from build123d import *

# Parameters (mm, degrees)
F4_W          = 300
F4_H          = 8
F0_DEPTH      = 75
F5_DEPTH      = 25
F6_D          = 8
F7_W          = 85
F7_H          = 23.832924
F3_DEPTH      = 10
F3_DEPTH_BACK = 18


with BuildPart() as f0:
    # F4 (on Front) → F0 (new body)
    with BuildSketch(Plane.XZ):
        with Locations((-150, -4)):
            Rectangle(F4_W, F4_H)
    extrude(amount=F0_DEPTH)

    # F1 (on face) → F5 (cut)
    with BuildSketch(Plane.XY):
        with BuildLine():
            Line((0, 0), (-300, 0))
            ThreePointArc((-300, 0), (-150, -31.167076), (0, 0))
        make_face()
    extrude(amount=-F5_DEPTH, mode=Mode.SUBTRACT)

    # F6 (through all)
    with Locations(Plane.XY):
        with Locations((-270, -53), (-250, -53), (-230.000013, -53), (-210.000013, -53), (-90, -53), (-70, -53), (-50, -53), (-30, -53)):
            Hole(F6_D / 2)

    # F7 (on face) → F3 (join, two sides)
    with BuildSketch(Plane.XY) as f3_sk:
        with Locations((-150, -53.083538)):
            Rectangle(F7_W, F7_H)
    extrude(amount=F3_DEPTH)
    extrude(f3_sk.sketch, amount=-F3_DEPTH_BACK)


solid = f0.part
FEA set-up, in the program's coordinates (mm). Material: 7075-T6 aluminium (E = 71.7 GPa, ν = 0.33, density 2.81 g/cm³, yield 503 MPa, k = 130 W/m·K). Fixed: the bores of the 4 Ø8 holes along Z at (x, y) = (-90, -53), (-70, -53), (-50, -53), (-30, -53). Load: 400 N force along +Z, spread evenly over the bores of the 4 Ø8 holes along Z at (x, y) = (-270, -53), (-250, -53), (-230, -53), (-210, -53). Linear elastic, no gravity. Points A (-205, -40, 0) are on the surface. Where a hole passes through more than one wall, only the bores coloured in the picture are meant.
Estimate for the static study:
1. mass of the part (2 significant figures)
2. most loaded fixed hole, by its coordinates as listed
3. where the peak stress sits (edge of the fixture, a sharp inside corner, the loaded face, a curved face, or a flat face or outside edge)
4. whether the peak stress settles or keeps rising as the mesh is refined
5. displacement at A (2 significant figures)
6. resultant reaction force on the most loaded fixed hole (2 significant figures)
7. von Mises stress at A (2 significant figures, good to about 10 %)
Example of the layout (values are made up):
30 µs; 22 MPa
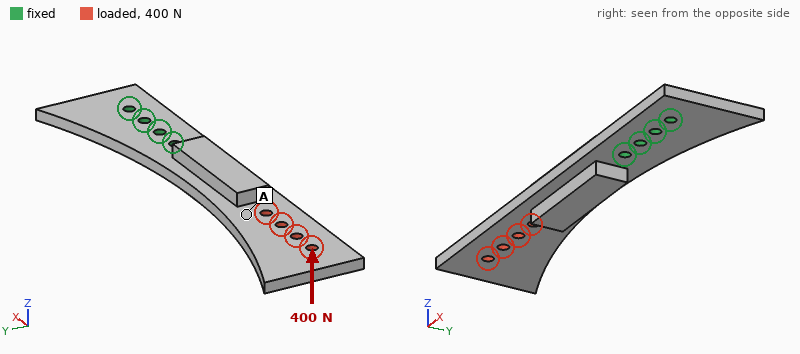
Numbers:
470 g; (-90, -53); edge of the fixture; keeps rising; 0.92 mm; 1.5 kN; 28 MPa
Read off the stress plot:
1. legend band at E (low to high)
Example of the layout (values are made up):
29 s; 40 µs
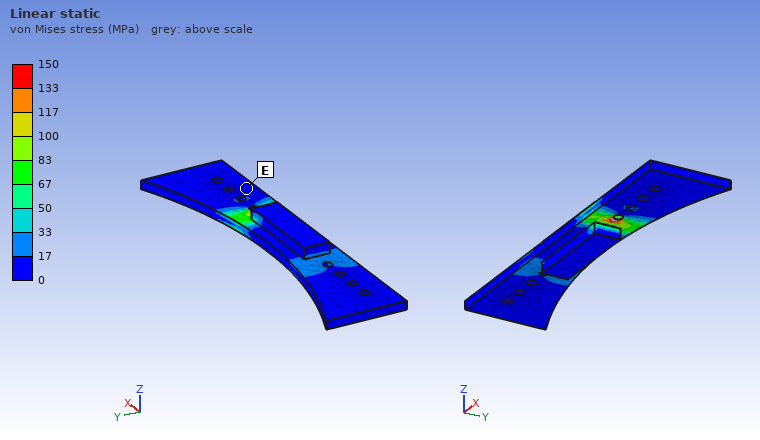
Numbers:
0 to 17 MPa
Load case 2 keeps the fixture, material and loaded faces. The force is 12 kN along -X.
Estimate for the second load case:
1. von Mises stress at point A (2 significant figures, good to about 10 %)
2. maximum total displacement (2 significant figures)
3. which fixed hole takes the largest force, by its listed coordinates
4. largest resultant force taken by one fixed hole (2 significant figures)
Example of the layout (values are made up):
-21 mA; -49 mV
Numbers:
30 MPa; 77 µm; (-90, -53); 8.6 kN
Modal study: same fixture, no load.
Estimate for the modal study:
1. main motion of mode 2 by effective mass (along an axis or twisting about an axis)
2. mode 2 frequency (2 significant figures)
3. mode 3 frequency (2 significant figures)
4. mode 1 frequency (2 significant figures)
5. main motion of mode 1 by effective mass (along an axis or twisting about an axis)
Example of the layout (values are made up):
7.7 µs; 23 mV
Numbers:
along Y; 640 Hz; 850 Hz; 190 Hz; along Z
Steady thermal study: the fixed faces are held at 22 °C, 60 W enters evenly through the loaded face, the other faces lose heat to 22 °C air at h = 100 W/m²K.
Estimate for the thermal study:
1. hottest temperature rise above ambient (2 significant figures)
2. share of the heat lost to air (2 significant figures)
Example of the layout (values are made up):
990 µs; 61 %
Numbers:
35 K; 86 %
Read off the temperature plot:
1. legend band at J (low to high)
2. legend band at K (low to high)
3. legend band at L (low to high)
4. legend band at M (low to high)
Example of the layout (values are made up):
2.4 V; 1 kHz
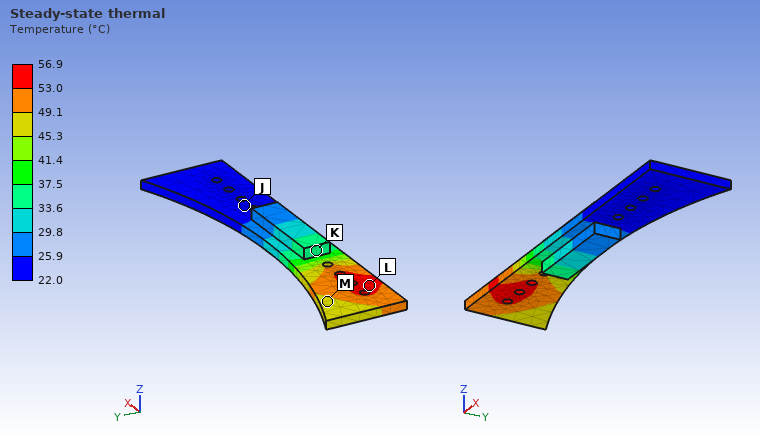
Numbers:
22.0 to 25.9 °C; 33.6 to 37.5 °C; 53.0 to 56.9 °C; 45.3 to 49.1 °C
